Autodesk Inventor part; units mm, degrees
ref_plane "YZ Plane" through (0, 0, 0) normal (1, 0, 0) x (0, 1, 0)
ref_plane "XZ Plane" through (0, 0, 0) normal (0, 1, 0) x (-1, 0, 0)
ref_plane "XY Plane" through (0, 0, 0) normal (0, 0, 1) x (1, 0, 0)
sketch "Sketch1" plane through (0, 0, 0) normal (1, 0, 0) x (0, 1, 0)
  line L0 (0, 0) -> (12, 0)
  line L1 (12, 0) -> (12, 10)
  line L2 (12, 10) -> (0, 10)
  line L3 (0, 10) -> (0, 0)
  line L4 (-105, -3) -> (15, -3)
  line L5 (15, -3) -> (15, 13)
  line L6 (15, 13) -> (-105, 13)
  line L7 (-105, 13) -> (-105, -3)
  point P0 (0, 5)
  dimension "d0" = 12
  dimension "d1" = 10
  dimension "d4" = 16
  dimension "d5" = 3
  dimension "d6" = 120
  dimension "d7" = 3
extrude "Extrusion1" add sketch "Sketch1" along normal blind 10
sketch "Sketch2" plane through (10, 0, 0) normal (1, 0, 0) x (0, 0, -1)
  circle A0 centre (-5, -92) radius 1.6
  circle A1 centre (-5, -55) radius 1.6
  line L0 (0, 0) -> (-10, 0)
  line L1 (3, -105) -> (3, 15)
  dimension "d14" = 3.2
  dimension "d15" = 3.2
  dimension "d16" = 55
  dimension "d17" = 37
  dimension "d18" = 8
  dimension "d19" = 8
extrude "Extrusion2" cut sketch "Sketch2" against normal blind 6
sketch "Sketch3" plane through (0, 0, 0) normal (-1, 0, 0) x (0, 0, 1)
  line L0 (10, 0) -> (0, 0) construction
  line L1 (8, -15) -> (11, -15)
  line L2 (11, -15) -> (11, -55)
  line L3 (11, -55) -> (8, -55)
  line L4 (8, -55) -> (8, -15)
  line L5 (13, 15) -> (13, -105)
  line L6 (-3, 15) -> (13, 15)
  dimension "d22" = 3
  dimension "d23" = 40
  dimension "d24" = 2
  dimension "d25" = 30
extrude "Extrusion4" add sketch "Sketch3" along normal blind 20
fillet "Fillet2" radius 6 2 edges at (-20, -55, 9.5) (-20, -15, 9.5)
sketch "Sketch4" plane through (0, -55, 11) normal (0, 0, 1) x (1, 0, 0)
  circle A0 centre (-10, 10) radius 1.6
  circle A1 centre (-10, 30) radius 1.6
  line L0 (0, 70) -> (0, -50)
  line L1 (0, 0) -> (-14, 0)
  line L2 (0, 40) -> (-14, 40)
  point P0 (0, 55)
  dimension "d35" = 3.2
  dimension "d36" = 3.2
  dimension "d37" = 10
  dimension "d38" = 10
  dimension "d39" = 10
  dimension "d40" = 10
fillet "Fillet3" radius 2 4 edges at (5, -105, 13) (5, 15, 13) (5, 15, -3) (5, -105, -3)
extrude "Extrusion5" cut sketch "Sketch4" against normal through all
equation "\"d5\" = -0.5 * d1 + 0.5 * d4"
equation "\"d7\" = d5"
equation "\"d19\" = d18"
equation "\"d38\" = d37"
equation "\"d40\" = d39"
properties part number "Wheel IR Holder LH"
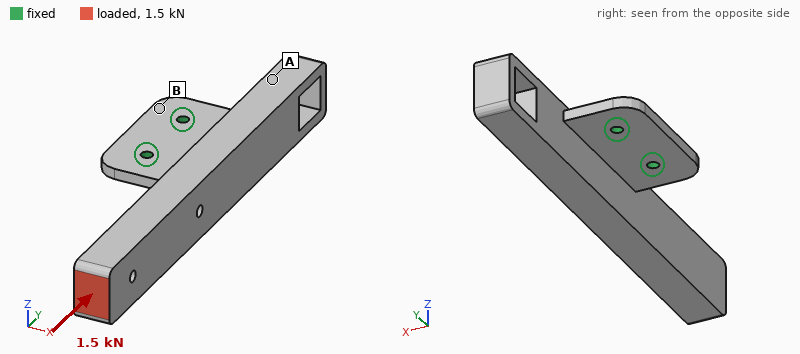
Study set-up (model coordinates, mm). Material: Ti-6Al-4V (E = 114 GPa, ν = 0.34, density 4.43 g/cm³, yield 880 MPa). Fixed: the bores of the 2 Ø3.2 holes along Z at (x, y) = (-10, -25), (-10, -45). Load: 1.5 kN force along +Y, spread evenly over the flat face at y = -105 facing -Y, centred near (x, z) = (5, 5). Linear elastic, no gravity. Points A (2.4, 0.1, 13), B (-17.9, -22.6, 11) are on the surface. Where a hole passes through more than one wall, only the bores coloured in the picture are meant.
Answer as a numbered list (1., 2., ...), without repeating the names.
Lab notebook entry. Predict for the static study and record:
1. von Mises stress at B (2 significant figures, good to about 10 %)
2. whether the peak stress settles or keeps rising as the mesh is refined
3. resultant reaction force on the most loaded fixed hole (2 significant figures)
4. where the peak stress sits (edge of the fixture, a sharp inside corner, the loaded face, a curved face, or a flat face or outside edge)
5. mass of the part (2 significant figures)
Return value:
1. 16 MPa
2. keeps rising
3. 1.3 kN
4. edge of the fixture
5. 89 g
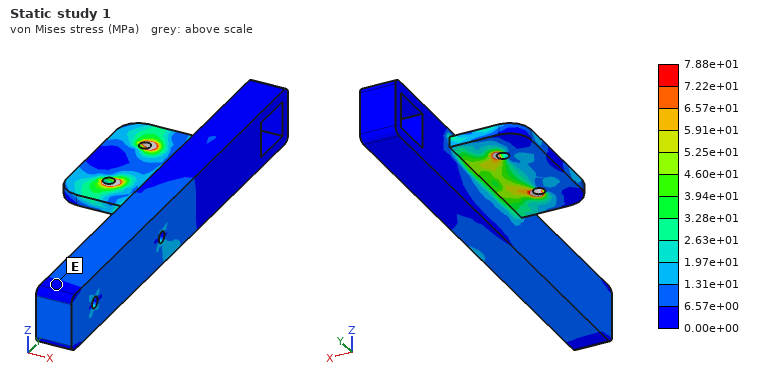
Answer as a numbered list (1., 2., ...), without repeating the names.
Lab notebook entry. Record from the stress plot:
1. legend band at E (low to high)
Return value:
1. 0.00e+00 to 6.57e+00 MPa
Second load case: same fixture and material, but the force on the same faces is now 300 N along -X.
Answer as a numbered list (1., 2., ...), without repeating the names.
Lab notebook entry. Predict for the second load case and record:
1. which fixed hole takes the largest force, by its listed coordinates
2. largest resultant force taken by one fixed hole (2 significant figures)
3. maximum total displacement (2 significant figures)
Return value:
1. (-10, -45)
2. 1.2 kN
3. 0.19 mm
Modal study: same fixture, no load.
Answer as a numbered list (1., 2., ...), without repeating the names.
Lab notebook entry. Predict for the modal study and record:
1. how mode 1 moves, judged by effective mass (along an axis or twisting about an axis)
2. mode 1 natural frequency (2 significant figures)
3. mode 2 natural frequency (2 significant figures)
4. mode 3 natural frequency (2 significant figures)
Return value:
1. along Z
2. 1100 Hz
3. 1600 Hz
4. 2100 Hz
